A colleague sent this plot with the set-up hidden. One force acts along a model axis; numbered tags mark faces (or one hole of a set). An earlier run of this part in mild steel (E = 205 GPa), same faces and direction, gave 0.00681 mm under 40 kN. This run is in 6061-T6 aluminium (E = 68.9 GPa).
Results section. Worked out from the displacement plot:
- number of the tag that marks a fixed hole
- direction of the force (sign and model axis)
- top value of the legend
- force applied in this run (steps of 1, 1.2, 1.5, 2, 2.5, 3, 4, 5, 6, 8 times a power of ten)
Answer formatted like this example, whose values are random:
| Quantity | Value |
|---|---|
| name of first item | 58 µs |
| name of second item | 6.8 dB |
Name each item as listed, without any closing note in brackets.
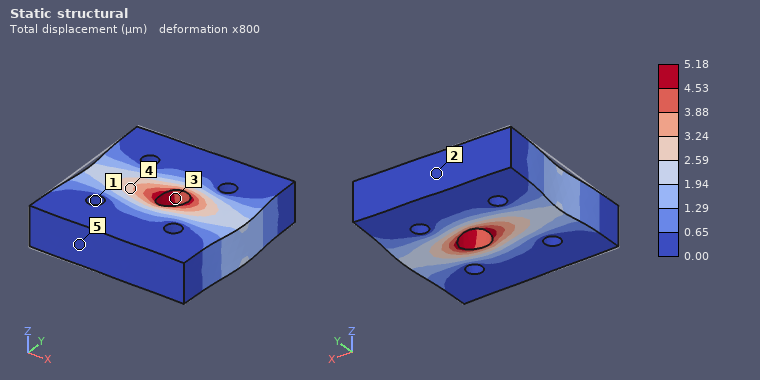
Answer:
| Quantity | Value |
|---|---|
| number of the tag that marks a fixed hole | 1 |
| direction of the force | +X |
| top value of the legend | 5.18 µm |
| force applied in this run | 10 kN |
